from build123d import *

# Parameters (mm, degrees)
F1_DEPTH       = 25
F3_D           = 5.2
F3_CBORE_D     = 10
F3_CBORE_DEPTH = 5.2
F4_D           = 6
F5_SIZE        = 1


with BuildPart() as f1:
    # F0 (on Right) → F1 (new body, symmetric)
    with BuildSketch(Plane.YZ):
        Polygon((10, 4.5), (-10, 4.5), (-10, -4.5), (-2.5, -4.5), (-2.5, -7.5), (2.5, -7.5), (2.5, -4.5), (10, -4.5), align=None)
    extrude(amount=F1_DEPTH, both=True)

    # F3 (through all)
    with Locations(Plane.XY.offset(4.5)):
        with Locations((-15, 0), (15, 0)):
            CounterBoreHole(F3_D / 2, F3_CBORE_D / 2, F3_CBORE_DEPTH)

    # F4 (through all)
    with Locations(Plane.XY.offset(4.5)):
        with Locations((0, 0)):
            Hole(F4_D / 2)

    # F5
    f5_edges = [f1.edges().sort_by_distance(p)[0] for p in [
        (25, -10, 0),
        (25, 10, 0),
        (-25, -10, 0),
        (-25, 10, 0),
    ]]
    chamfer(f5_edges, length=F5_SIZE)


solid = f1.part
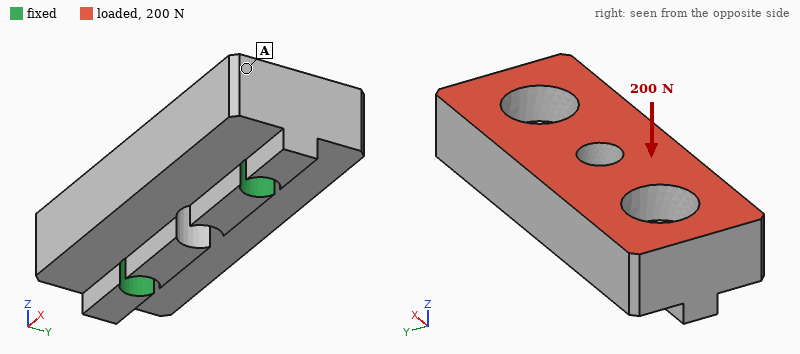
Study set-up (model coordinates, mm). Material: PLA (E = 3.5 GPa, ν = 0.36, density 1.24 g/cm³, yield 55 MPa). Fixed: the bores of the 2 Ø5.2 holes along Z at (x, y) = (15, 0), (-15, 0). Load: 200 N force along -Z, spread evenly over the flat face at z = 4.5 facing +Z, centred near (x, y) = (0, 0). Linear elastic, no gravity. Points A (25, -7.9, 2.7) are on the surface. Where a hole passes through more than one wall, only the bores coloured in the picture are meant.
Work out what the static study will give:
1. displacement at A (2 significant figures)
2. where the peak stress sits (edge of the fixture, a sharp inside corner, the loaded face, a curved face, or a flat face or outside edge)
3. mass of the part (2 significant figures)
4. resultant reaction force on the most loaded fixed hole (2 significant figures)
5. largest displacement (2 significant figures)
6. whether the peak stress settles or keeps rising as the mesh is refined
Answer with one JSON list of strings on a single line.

["4.2 µm", "edge of the fixture", "10 g", "100 N", "7.9 µm", "keeps rising"]
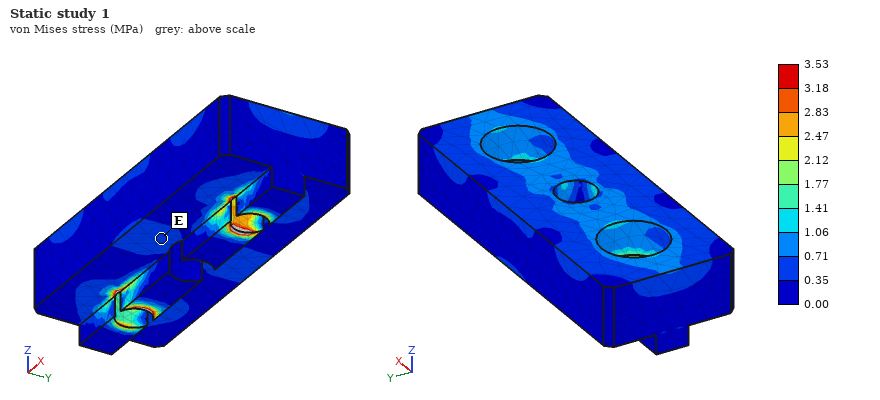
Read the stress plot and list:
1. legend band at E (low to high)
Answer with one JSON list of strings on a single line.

["0.35 to 0.71 MPa"]
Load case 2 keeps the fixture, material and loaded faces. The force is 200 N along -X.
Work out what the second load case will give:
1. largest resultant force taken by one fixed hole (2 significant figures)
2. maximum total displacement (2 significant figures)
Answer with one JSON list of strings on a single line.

["110 N", "11 µm"]
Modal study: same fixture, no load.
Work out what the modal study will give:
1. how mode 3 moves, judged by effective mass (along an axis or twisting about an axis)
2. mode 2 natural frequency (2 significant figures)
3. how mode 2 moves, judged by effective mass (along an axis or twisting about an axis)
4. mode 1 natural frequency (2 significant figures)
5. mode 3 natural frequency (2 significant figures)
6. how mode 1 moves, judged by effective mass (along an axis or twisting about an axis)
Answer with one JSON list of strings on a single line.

["along Z", "8300 Hz", "twisting about Z", "5600 Hz", "9200 Hz", "along Y"]
